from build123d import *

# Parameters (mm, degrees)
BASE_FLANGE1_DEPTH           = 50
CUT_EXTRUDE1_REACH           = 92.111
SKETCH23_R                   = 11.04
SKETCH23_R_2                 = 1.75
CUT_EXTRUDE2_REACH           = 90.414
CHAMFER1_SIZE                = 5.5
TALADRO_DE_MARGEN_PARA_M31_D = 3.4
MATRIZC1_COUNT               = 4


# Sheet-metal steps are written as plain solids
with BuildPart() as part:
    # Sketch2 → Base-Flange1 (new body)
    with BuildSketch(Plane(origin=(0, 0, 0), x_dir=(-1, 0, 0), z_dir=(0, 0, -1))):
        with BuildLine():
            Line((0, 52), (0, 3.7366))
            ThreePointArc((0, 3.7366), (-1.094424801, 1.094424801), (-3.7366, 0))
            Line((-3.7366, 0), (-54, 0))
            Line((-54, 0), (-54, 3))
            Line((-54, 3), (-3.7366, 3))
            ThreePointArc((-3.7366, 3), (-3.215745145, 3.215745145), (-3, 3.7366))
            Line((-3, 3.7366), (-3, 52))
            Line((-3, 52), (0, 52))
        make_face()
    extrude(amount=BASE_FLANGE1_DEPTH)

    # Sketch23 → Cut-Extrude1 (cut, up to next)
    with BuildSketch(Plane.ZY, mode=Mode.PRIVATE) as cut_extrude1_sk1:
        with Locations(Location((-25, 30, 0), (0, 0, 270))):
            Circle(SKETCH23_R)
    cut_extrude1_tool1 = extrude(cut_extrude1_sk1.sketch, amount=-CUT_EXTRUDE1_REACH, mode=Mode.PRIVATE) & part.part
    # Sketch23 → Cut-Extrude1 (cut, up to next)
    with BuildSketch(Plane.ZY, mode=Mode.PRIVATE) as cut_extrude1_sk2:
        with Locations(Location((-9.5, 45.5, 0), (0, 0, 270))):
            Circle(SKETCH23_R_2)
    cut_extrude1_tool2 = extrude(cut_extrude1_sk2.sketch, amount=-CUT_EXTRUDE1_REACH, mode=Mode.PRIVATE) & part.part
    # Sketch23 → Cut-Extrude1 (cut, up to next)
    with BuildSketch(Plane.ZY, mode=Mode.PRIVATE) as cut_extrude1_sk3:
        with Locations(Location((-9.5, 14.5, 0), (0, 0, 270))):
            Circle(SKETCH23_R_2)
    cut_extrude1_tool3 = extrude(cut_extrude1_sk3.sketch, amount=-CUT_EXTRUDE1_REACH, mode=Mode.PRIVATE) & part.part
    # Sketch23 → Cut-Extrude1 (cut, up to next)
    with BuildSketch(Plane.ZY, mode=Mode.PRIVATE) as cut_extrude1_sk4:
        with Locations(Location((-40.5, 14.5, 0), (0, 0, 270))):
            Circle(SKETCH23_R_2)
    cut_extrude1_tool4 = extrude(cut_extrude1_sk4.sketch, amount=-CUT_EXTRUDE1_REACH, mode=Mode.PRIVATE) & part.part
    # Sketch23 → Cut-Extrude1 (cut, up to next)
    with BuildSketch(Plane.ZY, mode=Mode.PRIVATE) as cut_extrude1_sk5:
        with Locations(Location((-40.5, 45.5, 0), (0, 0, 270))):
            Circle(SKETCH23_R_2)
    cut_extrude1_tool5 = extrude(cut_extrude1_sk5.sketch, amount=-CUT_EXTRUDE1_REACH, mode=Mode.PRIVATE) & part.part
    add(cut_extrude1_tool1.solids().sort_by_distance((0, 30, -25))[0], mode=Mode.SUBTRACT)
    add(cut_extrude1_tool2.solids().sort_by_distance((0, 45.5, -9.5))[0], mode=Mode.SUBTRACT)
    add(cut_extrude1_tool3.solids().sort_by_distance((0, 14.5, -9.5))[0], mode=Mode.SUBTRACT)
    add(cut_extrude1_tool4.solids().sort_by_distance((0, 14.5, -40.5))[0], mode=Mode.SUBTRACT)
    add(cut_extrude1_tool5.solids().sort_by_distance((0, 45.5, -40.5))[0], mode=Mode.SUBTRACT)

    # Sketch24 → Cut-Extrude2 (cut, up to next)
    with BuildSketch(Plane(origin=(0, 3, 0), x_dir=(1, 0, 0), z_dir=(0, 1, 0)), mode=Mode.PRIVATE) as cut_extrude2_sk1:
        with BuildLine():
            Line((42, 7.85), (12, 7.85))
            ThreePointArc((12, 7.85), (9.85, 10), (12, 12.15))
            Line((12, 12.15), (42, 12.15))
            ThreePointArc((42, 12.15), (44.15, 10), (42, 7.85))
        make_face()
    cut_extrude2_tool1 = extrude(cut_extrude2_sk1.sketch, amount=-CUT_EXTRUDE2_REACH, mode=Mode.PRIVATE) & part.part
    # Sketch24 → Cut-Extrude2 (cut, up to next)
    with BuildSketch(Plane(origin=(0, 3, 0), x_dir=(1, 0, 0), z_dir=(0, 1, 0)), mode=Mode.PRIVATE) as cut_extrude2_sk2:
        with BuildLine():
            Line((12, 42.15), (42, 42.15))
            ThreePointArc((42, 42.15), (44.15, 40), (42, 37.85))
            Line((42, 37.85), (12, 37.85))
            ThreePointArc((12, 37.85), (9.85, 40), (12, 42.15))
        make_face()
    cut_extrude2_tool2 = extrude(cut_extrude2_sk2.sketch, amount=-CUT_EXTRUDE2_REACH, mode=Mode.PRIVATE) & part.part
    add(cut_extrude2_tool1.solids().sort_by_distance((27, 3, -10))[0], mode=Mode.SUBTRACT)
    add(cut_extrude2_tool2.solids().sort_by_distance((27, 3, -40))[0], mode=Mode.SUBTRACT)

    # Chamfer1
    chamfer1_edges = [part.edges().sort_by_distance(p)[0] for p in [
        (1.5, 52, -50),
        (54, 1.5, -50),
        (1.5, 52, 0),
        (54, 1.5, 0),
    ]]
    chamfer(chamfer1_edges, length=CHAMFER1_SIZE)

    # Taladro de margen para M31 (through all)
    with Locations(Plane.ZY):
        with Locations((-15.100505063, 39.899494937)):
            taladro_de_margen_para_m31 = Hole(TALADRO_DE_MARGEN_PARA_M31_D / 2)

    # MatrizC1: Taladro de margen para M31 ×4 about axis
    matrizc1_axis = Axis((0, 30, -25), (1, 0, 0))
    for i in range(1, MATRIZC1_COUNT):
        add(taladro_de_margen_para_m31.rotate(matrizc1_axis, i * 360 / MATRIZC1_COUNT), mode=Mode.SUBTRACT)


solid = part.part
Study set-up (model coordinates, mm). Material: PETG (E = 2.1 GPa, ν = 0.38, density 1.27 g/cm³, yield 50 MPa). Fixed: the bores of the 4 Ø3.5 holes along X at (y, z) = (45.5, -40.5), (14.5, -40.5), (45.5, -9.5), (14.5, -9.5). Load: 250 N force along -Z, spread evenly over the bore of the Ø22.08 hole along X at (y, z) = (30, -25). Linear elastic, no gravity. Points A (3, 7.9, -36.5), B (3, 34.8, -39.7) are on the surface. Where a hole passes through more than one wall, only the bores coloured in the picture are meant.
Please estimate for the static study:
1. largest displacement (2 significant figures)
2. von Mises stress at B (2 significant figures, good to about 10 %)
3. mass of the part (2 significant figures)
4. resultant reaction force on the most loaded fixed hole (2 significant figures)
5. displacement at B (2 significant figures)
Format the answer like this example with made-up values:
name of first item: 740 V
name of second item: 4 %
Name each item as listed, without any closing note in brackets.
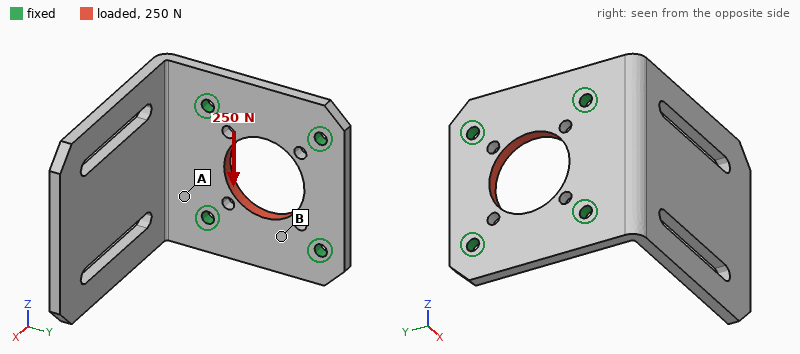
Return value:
largest displacement: 20 µm
von Mises stress at B: 1.0 MPa
mass of the part: 16 g
resultant reaction force on the most loaded fixed hole: 65 N
displacement at B: 16 µm
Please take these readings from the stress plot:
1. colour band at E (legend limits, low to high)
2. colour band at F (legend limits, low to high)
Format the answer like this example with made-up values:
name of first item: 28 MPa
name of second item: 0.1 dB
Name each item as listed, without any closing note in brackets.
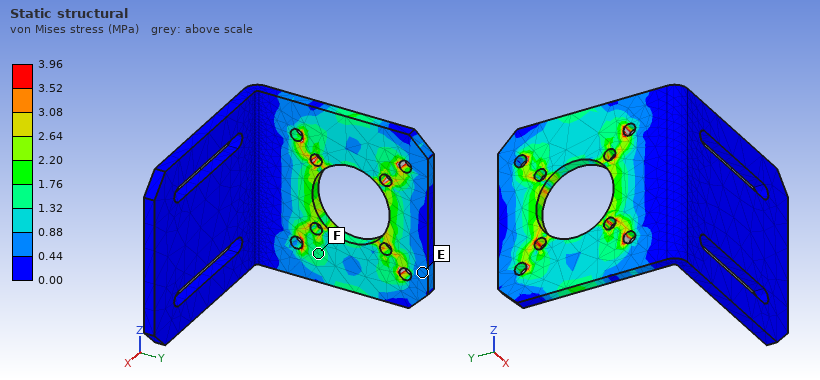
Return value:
colour band at E: 0.44 to 0.88 MPa
colour band at F: 1.32 to 1.76 MPa
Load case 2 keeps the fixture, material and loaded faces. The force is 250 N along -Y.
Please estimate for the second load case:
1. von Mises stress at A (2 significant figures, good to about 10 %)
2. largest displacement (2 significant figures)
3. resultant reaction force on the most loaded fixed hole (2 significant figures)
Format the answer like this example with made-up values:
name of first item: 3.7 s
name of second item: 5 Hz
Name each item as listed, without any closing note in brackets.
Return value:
von Mises stress at A: 1.1 MPa
largest displacement: 25 µm
resultant reaction force on the most loaded fixed hole: 64 N
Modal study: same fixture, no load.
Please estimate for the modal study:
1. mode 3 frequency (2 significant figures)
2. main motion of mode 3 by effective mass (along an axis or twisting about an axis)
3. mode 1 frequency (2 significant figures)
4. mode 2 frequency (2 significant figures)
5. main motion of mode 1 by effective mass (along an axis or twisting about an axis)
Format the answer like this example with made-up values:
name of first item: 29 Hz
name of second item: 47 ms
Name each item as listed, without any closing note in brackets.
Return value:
mode 3 frequency: 640 Hz
main motion of mode 3 by effective mass: along Z
mode 1 frequency: 170 Hz
mode 2 frequency: 450 Hz
main motion of mode 1 by effective mass: along Y
